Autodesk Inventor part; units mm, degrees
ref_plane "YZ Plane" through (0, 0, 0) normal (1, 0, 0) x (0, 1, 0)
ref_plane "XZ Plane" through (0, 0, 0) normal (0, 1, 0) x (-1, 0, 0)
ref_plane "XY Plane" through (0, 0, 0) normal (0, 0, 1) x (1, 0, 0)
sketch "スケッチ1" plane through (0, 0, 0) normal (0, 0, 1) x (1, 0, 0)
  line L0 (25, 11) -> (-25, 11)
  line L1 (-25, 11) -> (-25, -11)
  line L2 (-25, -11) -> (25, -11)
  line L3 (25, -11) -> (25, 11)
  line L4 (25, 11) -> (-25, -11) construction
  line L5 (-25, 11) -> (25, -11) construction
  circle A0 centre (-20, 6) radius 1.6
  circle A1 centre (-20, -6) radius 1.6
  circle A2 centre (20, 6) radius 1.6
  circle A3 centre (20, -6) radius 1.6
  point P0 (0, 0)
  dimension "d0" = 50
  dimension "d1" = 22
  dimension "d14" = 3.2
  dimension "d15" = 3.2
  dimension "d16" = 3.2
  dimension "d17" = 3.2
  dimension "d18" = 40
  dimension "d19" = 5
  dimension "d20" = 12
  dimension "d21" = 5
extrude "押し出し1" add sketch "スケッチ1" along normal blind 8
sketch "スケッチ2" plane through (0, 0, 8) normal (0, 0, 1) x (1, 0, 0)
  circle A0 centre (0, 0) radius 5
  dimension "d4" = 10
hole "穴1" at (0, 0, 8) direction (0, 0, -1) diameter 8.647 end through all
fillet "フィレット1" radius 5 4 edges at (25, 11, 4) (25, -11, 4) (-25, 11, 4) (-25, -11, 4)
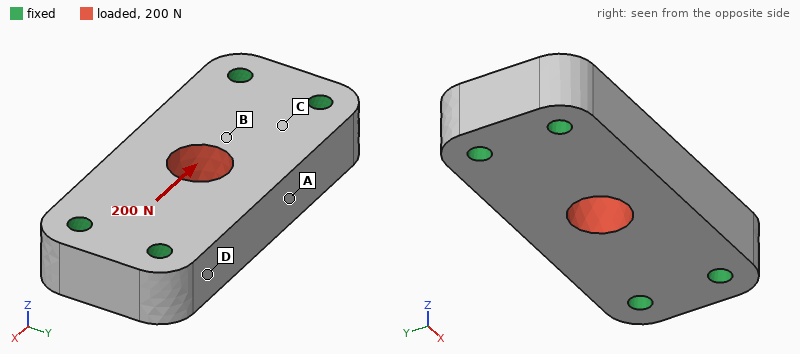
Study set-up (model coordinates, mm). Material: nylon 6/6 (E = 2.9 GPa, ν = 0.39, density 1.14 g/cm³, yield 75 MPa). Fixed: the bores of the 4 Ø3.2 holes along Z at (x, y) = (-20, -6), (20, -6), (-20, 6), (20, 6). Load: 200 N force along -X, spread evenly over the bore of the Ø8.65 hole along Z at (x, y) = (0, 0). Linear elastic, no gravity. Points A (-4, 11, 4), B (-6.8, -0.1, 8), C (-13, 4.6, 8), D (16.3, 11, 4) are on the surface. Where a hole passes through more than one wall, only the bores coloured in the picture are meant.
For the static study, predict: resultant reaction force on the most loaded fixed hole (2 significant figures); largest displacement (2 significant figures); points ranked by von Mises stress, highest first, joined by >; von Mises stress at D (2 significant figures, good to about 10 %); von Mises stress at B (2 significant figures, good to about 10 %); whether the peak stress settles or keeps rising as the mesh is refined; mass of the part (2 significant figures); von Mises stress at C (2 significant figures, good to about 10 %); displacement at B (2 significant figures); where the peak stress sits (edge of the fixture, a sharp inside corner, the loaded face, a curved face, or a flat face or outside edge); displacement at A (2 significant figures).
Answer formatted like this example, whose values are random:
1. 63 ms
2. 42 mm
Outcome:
1. 51 N
2. 4.8 µm
3. B > C > D > A
4. 0.29 MPa
5. 0.96 MPa
6. keeps rising
7. 9.0 g
8. 0.72 MPa
9. 3.5 µm
10. edge of the fixture
11. 2.3 µm
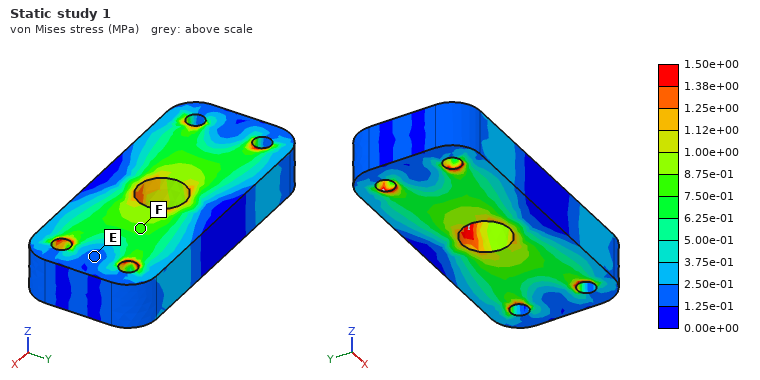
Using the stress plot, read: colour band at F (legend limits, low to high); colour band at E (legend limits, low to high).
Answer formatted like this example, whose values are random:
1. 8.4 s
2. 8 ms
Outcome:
1. 7.50e-01 to 8.75e-01 MPa
2. 1.25e-01 to 2.50e-01 MPa
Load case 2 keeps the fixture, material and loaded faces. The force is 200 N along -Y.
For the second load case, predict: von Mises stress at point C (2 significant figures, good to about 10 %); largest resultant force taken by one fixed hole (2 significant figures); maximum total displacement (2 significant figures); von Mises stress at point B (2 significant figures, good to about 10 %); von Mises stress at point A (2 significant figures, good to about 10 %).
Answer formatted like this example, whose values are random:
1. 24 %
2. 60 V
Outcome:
1. 1.3 MPa
2. 78 N
3. 16 µm
4. 1.6 MPa
5. 1.4 MPa
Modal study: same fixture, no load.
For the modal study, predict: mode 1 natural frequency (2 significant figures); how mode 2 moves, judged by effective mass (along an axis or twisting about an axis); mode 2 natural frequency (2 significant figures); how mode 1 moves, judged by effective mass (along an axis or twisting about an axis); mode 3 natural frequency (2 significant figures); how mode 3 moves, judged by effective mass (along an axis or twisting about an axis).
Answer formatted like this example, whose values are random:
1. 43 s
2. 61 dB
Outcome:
1. 6800 Hz
2. twisting about X
3. 8900 Hz
4. along Z
5. 10 kHz
6. along Y
